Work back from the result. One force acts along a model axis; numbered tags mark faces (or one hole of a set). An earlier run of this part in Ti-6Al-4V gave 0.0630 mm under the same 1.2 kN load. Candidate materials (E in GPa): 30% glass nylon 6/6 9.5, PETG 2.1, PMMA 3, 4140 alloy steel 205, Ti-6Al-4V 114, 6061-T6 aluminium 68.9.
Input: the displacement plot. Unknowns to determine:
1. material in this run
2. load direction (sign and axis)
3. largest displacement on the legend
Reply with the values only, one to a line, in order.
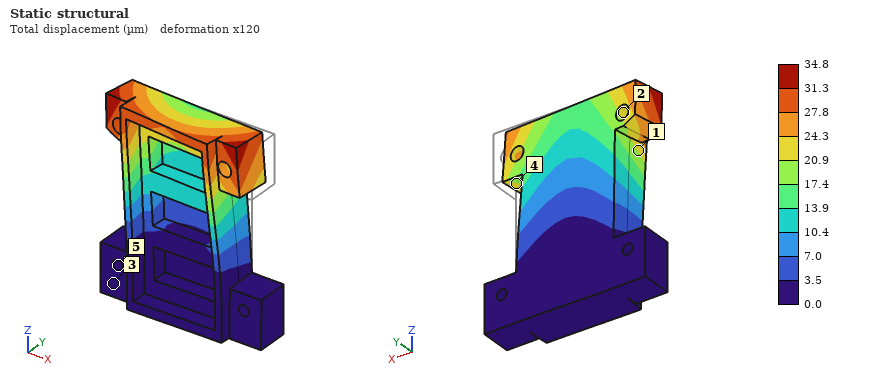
4140 alloy steel
-X
34.8 µm
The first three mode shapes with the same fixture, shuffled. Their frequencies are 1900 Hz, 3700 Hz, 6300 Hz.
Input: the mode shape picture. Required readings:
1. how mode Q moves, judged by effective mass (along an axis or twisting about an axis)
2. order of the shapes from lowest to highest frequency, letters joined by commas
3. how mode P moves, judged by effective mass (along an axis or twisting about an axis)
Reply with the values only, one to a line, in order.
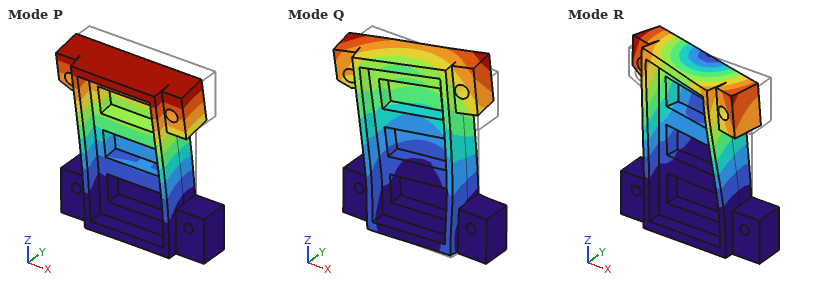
along X
P, R, Q
along Y
